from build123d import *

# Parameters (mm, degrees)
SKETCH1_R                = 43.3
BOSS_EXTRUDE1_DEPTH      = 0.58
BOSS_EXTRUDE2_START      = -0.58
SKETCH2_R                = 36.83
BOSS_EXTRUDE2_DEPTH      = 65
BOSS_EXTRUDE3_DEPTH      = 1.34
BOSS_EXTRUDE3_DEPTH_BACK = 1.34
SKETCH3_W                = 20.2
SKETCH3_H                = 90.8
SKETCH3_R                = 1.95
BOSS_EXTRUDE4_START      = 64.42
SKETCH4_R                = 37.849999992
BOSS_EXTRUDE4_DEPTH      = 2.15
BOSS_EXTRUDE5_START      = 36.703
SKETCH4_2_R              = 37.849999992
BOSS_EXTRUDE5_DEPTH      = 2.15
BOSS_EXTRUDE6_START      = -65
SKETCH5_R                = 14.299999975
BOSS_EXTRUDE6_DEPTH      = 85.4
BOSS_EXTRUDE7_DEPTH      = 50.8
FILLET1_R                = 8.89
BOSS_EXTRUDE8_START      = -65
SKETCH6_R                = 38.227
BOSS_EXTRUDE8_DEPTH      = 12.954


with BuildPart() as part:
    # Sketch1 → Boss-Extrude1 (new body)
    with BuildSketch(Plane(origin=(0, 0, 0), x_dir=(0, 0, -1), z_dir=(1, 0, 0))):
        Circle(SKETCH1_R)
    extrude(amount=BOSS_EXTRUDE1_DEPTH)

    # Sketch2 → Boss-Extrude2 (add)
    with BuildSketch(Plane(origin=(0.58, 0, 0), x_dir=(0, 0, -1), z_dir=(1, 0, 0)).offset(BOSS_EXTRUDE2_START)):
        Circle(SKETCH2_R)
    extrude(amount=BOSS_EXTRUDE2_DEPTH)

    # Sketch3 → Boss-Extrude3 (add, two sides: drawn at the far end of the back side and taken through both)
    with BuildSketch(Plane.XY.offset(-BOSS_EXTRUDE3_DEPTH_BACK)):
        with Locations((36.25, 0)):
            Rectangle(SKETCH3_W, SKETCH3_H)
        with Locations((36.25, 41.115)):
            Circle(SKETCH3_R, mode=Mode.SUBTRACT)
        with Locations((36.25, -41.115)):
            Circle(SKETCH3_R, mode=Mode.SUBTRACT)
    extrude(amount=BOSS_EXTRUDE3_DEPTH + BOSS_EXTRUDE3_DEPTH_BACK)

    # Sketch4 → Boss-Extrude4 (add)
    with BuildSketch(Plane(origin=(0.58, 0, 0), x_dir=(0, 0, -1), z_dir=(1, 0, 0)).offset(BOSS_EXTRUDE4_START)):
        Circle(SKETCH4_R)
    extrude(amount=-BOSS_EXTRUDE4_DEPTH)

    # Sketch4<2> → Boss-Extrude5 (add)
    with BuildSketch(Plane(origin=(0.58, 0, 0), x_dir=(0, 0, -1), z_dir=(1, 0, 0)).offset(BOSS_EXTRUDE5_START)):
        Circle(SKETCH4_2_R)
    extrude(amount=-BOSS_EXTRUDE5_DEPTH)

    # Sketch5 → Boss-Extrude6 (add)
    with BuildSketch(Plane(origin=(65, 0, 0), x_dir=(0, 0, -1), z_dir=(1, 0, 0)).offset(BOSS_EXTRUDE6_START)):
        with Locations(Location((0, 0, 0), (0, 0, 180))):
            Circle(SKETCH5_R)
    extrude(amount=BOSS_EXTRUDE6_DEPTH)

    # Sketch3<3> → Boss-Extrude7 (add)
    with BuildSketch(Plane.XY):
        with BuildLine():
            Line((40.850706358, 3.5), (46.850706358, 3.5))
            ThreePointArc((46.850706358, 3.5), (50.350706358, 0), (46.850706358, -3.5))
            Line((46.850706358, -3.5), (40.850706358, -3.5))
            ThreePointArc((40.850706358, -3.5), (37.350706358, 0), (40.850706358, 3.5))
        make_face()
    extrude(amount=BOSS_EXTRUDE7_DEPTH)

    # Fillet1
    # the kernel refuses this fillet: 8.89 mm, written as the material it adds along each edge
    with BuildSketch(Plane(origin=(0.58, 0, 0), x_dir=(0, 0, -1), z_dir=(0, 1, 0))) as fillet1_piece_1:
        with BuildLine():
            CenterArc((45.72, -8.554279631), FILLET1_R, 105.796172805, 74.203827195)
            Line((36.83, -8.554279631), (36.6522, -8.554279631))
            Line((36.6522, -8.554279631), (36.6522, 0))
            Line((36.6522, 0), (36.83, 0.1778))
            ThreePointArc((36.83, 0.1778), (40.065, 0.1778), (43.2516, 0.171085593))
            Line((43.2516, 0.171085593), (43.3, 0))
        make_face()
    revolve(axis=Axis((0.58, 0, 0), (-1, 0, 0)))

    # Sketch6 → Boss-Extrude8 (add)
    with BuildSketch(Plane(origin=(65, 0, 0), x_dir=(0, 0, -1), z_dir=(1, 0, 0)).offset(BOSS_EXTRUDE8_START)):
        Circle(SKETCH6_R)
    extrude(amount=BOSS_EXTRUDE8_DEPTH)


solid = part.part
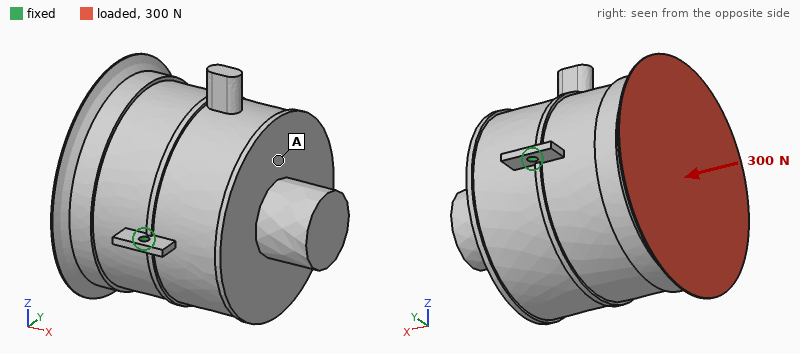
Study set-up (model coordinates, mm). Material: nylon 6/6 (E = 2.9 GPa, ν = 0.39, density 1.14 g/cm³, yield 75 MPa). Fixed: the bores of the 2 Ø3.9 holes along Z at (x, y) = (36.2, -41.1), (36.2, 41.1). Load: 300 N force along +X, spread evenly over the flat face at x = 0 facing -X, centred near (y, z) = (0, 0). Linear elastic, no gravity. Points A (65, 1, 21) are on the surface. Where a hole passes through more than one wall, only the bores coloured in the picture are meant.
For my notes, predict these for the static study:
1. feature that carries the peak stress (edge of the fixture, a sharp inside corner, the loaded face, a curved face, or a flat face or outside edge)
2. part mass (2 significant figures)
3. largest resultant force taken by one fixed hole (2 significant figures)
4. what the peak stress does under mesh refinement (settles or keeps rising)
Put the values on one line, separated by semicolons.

edge of the fixture; 340 g; 150 N; keeps rising
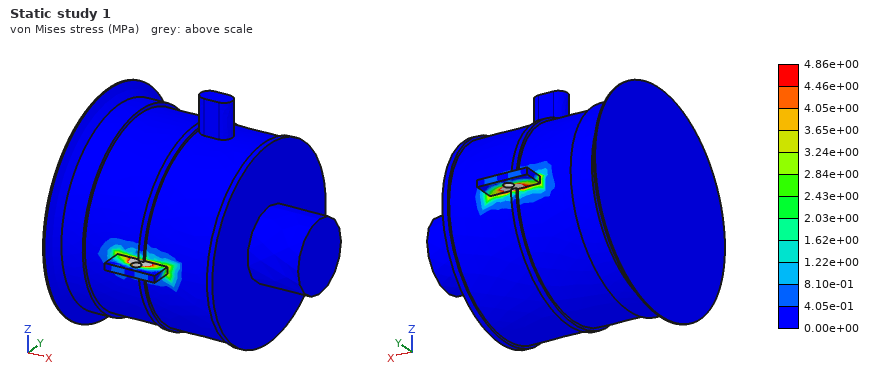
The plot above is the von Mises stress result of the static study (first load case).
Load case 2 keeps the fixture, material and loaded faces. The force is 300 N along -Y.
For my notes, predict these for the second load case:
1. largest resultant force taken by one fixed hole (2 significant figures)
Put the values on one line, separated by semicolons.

200 N
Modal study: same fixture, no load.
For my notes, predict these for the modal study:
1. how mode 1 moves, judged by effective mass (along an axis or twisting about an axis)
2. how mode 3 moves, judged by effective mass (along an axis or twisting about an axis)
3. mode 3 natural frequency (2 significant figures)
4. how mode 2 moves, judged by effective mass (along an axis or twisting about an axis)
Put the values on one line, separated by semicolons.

twisting about Y; along X; 1100 Hz; along Z
